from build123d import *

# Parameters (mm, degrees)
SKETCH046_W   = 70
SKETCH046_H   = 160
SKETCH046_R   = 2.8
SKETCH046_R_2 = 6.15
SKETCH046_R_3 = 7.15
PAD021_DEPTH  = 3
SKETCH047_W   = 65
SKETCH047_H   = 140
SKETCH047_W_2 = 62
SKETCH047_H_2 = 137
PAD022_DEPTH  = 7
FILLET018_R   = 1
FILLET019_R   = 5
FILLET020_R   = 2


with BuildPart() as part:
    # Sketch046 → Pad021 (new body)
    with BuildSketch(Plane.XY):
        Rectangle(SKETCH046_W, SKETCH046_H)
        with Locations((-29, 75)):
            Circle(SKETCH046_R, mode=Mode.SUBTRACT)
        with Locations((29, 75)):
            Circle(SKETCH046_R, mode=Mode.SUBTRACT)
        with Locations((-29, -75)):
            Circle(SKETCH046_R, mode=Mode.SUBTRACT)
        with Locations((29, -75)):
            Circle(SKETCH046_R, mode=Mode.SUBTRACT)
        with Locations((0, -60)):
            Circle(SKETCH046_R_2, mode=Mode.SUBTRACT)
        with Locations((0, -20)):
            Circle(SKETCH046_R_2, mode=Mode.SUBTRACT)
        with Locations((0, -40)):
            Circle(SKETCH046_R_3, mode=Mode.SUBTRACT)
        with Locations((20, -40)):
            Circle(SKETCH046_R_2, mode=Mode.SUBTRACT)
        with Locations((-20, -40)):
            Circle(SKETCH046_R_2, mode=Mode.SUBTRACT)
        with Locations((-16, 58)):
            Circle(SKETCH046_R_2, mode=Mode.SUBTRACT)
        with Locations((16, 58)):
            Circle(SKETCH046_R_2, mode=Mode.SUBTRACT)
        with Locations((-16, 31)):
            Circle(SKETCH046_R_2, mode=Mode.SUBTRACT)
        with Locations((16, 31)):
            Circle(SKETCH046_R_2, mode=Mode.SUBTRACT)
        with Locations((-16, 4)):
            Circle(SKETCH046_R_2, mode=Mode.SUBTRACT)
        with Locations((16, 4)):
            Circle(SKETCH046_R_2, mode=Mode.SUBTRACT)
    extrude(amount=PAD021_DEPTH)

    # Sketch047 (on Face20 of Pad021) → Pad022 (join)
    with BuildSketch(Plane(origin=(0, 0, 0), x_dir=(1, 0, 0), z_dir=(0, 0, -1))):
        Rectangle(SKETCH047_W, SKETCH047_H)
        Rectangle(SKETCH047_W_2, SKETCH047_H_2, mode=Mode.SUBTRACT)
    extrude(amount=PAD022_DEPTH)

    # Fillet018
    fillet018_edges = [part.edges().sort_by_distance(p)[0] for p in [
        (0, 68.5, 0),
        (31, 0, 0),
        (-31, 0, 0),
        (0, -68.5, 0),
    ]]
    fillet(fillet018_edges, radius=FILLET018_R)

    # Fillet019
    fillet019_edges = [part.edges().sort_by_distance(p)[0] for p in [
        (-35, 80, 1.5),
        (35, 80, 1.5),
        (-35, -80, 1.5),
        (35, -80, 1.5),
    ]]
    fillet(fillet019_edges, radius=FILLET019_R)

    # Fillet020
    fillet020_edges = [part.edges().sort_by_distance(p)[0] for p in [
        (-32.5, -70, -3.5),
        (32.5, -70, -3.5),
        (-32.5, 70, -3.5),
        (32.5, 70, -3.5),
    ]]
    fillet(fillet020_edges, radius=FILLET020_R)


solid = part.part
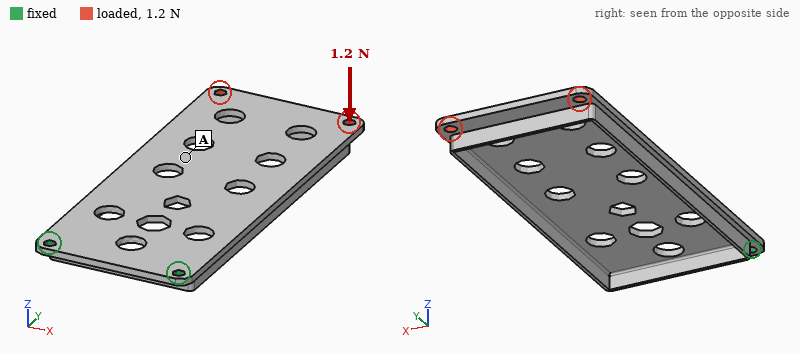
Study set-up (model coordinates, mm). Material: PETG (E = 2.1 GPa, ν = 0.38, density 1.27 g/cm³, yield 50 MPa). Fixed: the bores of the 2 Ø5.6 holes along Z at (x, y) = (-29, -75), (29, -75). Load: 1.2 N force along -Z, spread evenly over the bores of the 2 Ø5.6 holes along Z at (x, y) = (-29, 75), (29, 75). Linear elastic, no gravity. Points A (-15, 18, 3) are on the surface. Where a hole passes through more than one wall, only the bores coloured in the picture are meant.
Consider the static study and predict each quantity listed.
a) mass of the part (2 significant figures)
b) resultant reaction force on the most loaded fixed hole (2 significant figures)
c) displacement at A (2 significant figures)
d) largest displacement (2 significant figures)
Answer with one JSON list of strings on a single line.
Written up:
["43 g", "4.0 N", "0.90 mm", "1.8 mm"]
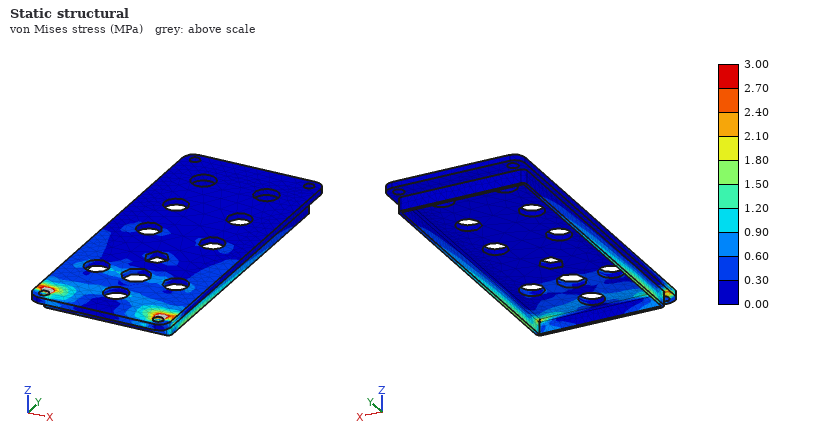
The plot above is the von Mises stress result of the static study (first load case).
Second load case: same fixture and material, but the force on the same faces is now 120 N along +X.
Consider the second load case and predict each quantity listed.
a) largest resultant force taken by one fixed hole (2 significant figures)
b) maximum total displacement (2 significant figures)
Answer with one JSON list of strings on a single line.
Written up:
["310 N", "1.2 mm"]
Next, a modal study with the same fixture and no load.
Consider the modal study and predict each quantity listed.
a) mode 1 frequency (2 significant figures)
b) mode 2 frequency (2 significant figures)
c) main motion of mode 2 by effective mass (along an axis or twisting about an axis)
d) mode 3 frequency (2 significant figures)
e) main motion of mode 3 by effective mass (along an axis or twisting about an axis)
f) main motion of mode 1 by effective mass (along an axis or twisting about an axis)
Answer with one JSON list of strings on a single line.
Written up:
["37 Hz", "120 Hz", "twisting about Y", "270 Hz", "along Z", "along Z"]
